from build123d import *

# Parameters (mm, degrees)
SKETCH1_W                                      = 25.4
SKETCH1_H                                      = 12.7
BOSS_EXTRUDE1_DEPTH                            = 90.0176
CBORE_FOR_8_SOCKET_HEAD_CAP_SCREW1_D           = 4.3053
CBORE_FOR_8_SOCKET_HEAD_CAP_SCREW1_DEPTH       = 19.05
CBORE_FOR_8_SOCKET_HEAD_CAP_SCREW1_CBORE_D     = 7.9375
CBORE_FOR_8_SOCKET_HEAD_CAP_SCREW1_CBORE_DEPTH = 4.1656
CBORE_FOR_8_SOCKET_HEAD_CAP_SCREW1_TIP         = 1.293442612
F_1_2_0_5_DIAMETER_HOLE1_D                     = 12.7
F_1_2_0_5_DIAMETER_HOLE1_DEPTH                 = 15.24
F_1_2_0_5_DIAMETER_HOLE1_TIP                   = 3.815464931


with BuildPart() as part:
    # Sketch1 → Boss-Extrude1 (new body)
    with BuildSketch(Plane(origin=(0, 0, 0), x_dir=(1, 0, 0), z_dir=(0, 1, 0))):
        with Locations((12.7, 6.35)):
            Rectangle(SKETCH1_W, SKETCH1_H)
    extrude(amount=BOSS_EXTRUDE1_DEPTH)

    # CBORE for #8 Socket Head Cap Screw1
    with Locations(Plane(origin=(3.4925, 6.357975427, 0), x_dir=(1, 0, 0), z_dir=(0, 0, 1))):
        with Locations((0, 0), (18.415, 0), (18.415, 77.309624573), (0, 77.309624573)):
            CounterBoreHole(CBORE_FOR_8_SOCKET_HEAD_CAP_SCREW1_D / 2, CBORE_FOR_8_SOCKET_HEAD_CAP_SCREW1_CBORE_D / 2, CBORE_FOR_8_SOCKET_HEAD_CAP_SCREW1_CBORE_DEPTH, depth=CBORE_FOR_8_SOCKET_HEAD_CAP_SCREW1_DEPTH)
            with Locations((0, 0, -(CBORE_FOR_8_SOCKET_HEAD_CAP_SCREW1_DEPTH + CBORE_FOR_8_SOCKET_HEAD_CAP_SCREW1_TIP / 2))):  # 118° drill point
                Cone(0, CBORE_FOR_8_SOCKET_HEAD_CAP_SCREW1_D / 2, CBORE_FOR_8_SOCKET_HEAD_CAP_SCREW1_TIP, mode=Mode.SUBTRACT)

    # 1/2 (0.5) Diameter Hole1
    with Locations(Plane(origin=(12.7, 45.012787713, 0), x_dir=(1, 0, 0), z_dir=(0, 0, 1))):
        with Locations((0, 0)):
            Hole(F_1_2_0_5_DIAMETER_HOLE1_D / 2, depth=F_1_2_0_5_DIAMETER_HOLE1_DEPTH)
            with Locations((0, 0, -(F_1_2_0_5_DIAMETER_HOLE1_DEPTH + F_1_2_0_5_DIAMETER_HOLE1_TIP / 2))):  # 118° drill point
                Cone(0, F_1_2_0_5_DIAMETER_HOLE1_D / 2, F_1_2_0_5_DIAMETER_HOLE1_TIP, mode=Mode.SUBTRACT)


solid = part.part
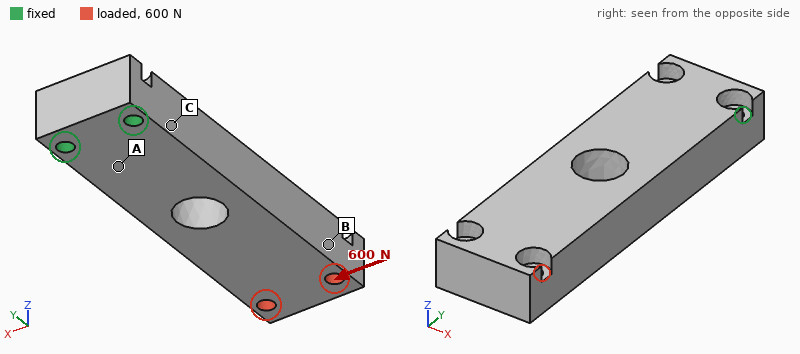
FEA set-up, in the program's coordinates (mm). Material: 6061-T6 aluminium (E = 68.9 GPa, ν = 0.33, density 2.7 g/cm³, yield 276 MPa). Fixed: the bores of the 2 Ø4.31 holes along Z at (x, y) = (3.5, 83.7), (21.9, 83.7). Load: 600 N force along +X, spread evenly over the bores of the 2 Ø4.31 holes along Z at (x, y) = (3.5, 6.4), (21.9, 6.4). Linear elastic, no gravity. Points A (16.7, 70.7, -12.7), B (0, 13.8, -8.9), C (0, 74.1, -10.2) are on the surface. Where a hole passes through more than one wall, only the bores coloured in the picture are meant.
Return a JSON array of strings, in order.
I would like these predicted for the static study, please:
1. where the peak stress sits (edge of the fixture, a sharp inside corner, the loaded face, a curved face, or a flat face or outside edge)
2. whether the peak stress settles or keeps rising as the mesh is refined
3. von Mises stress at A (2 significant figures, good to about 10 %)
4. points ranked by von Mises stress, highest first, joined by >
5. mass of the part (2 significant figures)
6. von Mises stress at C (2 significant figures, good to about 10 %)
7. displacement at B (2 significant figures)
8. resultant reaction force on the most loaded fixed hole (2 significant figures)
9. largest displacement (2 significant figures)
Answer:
["edge of the fixture", "keeps rising", "15 MPa", "C > A > B", "71 g", "35 MPa", "0.086 mm", "2.4 kN", "0.11 mm"]
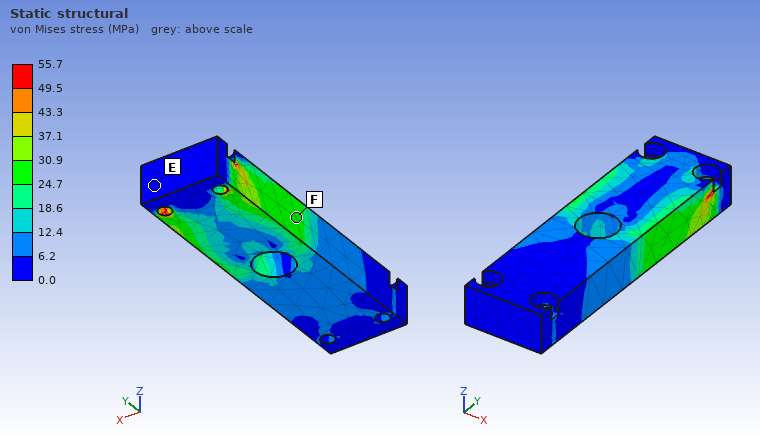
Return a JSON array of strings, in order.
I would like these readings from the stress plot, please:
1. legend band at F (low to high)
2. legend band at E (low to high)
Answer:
["24.7 to 30.9 MPa", "0.0 to 6.2 MPa"]
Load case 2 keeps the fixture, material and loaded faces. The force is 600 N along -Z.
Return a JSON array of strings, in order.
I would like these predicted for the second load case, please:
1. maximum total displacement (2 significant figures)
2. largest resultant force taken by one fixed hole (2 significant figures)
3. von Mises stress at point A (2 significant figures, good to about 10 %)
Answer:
["0.53 mm", "380 N", "57 MPa"]
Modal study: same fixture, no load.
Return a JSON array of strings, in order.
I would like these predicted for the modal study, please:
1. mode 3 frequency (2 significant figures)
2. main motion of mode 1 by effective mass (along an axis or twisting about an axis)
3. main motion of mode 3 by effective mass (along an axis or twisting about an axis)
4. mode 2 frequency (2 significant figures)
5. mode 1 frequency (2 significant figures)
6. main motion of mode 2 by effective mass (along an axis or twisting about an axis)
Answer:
["6600 Hz", "along Z", "twisting about Y", "2700 Hz", "1200 Hz", "along X"]
